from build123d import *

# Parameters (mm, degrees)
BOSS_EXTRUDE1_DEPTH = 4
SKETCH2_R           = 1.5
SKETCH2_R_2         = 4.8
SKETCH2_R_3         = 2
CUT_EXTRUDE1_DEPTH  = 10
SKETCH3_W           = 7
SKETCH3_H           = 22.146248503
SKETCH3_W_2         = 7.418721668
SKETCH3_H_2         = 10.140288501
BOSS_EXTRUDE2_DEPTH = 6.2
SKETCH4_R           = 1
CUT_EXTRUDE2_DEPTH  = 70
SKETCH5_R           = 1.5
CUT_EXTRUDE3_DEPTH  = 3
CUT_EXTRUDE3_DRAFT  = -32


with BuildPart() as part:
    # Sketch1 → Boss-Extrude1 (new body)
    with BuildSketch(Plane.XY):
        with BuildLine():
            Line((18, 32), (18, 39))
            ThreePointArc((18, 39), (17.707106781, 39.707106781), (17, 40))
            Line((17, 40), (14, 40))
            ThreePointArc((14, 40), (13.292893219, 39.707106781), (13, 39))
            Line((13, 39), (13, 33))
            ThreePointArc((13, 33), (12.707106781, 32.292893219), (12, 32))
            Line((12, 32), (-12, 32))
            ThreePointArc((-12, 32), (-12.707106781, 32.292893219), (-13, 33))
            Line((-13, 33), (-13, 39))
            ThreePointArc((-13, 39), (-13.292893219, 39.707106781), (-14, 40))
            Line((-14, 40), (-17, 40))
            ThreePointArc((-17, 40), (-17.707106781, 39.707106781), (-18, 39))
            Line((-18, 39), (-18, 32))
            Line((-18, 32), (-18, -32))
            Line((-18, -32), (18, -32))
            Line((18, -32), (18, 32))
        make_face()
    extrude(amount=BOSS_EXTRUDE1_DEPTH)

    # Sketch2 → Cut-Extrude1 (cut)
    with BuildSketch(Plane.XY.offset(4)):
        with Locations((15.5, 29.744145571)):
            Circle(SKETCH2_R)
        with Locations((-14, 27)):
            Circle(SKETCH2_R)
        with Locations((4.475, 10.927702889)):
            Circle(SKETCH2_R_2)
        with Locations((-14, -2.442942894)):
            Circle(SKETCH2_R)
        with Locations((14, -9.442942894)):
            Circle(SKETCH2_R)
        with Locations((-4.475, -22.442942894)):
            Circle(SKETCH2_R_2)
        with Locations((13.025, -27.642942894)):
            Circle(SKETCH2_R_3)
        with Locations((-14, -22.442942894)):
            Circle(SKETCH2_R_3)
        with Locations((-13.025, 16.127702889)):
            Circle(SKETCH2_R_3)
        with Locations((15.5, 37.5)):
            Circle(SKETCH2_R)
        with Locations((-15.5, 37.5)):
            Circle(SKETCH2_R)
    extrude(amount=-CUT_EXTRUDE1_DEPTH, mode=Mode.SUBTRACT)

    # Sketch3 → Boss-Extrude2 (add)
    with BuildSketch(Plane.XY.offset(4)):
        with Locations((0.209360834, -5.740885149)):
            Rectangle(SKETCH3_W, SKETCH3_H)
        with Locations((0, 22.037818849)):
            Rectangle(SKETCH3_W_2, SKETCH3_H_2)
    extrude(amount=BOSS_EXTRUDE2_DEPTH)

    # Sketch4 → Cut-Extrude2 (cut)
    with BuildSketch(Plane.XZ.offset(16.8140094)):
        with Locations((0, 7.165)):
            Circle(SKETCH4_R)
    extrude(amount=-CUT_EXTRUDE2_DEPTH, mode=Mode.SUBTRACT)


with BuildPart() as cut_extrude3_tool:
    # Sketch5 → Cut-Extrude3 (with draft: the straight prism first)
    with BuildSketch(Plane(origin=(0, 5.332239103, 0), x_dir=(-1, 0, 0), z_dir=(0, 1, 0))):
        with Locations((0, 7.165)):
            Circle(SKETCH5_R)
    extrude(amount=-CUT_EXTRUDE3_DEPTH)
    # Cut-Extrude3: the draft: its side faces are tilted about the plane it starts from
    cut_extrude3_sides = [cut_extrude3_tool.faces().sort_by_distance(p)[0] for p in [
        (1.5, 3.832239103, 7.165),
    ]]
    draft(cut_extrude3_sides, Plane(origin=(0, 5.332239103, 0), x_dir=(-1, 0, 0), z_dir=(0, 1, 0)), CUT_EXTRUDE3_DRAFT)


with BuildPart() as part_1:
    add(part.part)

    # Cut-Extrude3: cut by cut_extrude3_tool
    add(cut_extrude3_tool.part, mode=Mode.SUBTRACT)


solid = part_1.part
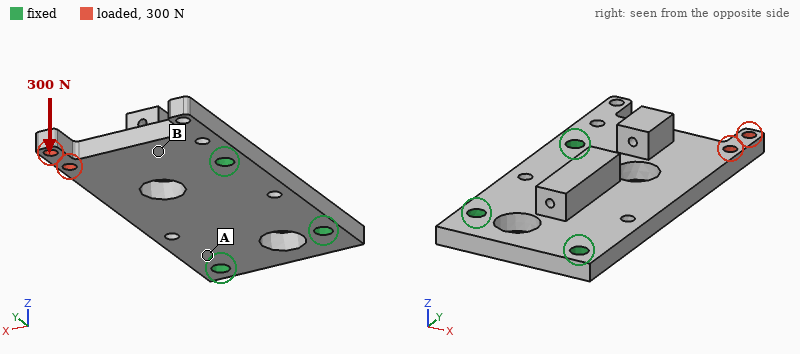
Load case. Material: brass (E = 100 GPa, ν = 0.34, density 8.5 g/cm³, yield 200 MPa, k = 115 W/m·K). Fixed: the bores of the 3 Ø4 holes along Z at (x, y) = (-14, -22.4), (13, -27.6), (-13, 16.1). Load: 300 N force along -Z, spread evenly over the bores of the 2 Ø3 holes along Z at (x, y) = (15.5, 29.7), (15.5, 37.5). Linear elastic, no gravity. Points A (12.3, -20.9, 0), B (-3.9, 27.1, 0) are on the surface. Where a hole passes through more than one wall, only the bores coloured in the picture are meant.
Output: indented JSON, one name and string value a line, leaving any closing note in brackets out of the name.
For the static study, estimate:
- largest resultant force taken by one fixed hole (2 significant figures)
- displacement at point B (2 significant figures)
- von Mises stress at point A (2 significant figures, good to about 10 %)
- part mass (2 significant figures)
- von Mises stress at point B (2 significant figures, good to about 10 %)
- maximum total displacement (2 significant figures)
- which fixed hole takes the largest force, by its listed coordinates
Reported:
{
  "largest resultant force taken by one fixed hole": "360 N",
  "displacement at point B": "0.054 mm",
  "von Mises stress at point A": "22 MPa",
  "part mass": "85 g",
  "von Mises stress at point B": "53 MPa",
  "maximum total displacement": "0.33 mm",
  "which fixed hole takes the largest force, by its listed coordinates": "(-13, 16.1)"
}
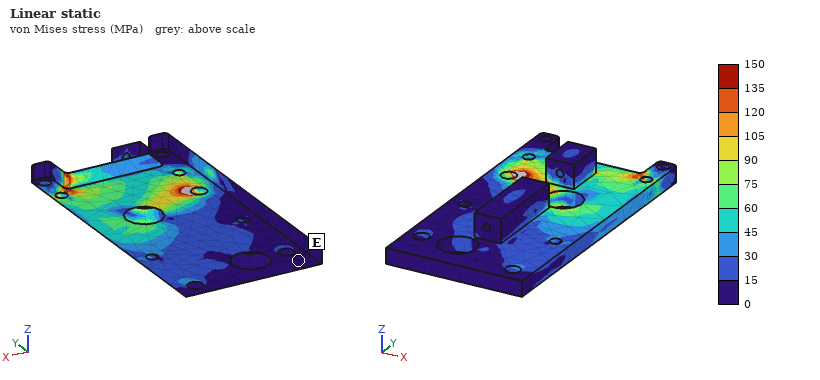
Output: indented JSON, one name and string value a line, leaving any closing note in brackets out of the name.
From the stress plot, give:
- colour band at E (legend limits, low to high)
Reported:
{
  "colour band at E": "0 to 15 MPa"
}
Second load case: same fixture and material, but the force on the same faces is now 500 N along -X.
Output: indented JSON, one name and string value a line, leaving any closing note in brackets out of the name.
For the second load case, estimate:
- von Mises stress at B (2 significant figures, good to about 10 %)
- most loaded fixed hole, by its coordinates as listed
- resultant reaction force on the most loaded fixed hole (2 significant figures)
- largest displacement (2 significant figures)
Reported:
{
  "von Mises stress at B": "12 MPa",
  "most loaded fixed hole, by its coordinates as listed": "(-13, 16.1)",
  "resultant reaction force on the most loaded fixed hole": "630 N",
  "largest displacement": "34 µm"
}
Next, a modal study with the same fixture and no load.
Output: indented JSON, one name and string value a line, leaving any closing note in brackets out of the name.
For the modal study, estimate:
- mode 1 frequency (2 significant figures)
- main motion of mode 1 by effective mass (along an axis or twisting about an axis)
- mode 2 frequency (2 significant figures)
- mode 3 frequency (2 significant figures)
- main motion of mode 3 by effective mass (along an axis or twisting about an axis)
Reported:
{
  "mode 1 frequency": "2300 Hz",
  "main motion of mode 1 by effective mass": "along Z",
  "mode 2 frequency": "4500 Hz",
  "mode 3 frequency": "7000 Hz",
  "main motion of mode 3 by effective mass": "along Z"
}
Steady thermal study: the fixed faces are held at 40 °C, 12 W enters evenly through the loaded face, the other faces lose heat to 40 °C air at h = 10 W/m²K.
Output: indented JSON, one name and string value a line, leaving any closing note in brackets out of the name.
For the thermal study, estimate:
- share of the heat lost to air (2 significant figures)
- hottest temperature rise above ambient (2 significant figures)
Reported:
{
  "share of the heat lost to air": "4.4 %",
  "hottest temperature rise above ambient": "71 K"
}
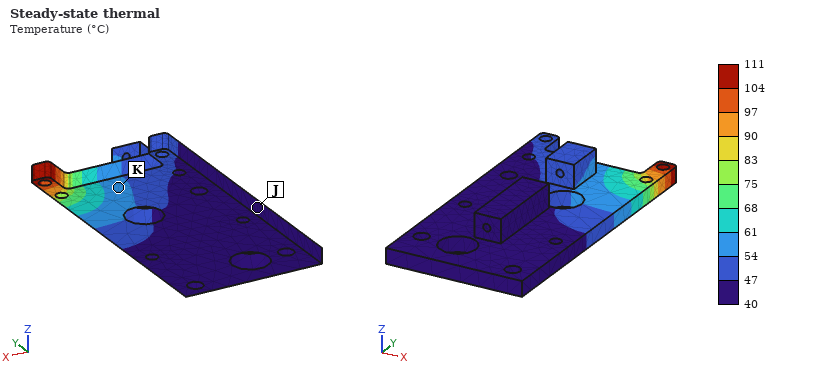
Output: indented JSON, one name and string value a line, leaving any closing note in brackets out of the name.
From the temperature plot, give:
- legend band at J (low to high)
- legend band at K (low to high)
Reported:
{
  "legend band at J": "40 to 47 °C",
  "legend band at K": "54 to 61 °C"
}
